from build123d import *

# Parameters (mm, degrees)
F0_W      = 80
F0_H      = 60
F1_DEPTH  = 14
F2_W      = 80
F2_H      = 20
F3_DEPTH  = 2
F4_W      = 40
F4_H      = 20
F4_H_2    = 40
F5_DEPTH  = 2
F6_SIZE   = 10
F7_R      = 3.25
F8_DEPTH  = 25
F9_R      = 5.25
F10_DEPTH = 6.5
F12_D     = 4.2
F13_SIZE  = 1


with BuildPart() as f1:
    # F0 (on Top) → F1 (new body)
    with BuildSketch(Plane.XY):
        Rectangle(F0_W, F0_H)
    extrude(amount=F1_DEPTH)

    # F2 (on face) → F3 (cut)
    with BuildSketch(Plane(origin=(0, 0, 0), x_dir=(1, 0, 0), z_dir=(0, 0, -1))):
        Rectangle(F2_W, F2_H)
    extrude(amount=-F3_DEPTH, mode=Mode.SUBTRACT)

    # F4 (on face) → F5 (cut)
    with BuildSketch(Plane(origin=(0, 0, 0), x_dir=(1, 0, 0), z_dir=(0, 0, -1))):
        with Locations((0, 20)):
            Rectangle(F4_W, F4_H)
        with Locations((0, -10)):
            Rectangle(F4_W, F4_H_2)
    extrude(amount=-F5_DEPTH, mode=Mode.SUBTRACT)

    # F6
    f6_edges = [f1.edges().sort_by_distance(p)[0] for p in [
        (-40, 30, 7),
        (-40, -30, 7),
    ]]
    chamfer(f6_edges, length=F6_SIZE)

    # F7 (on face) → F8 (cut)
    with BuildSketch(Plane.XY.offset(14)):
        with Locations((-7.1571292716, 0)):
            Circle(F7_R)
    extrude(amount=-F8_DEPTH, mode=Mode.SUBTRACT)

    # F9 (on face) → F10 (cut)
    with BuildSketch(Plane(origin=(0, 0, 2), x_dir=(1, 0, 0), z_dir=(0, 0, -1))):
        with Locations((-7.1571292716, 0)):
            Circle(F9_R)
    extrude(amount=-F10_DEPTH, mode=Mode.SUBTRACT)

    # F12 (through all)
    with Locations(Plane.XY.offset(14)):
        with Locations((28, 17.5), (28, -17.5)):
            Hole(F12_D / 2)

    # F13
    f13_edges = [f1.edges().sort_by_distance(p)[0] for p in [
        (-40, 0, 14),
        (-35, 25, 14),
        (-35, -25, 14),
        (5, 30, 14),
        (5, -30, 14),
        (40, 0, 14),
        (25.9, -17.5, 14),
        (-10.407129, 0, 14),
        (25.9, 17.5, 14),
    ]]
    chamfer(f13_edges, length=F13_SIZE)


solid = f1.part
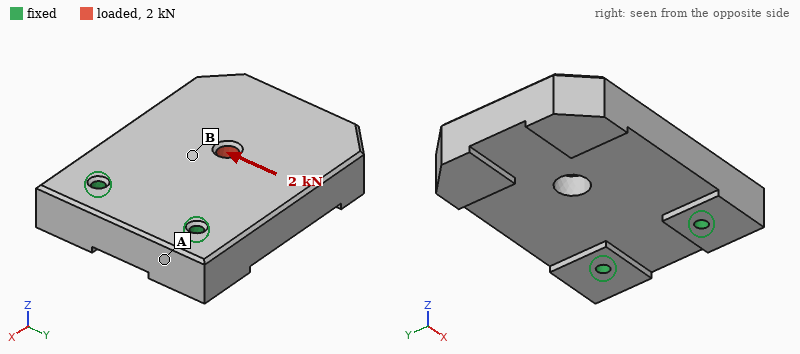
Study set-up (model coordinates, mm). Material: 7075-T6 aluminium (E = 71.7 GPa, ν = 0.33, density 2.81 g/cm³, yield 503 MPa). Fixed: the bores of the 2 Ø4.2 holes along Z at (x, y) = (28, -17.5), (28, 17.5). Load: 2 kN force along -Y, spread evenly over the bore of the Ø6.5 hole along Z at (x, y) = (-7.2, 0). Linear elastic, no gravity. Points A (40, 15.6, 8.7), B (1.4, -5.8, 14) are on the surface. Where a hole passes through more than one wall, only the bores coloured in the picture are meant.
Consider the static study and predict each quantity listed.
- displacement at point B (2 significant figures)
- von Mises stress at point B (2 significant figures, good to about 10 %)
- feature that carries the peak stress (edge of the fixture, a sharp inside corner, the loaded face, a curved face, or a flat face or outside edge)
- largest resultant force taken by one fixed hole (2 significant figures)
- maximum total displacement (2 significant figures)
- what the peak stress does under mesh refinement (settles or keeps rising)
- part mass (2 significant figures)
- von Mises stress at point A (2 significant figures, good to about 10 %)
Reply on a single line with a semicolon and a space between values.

6.2 µm; 10 MPa; edge of the fixture; 2.1 kN; 13 µm; keeps rising; 160 g; 4.8 MPa
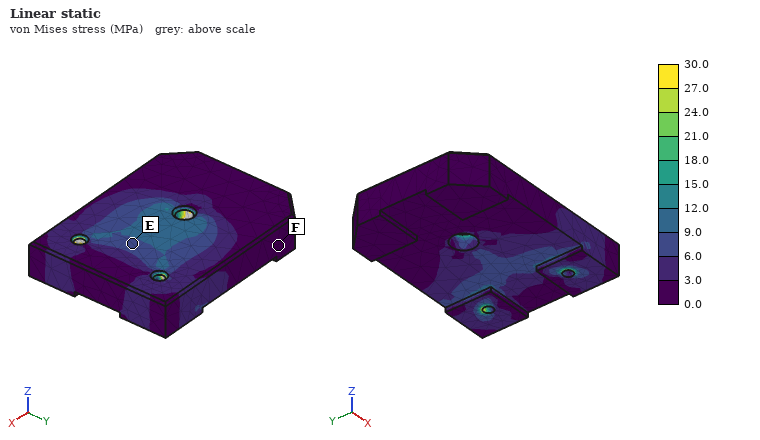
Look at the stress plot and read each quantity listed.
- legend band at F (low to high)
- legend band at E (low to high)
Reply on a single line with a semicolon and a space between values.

0.0 to 3.0 MPa; 6.0 to 9.0 MPa
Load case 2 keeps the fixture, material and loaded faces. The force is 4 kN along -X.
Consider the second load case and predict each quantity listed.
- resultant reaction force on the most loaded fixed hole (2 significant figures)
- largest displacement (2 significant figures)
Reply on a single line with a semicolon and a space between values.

2.0 kN; 38 µm
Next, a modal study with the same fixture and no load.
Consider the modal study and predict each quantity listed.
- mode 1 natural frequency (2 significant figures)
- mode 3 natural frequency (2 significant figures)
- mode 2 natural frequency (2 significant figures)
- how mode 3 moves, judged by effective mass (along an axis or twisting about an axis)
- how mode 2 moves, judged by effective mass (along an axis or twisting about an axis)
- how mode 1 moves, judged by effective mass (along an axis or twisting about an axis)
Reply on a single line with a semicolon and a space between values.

2000 Hz; 6300 Hz; 5100 Hz; along Y; twisting about X; along Z
